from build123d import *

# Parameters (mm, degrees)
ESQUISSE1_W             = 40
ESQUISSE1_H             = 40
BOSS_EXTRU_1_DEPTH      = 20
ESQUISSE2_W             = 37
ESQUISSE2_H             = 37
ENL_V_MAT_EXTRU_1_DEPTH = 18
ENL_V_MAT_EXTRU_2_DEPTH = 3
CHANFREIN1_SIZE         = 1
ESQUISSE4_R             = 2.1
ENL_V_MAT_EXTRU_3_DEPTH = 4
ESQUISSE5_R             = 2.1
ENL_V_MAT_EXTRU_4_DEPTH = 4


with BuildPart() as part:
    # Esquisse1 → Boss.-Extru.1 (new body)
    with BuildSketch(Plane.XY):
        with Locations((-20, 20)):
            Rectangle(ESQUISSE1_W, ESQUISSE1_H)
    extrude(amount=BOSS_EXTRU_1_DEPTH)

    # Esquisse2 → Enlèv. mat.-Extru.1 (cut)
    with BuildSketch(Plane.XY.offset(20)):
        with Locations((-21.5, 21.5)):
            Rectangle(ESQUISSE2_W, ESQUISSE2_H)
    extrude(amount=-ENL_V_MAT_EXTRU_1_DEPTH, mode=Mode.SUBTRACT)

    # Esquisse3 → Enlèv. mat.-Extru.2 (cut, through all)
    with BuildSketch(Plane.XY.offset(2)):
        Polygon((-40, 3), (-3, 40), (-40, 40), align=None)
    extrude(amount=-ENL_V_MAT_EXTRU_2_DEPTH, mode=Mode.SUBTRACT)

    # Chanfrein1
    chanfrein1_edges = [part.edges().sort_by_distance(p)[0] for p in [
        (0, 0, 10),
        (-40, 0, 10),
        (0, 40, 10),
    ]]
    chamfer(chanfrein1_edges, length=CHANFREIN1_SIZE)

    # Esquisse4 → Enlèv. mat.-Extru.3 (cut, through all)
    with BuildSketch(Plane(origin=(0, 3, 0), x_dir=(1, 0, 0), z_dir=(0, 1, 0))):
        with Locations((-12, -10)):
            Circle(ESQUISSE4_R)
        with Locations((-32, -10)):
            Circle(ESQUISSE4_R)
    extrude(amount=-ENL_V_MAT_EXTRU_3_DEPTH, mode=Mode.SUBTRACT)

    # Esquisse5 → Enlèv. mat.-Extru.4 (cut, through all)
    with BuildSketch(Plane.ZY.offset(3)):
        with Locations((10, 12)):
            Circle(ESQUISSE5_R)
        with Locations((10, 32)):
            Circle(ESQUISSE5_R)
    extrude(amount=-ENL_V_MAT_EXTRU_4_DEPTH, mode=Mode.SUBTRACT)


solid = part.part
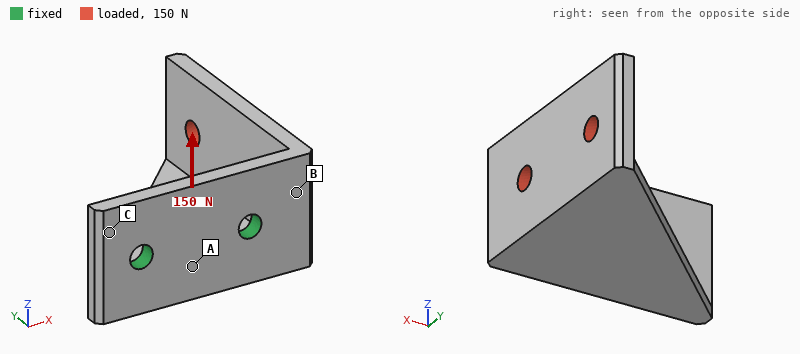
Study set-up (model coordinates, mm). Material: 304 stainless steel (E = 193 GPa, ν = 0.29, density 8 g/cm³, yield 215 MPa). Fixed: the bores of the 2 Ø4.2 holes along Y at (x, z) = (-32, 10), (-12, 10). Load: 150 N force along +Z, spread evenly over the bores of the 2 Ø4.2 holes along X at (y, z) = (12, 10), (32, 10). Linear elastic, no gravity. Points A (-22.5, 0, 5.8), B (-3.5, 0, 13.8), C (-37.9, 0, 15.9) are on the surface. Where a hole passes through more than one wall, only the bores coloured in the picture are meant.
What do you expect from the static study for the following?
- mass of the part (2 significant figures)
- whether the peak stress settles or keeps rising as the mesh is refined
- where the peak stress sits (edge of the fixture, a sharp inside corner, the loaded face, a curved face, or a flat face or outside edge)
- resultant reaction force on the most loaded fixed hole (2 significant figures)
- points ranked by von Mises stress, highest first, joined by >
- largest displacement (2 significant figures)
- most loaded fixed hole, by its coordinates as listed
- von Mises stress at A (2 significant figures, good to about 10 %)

46 g
keeps rising
edge of the fixture
200 N
B > A > C
56 µm
(-12, 10)
18 MPa
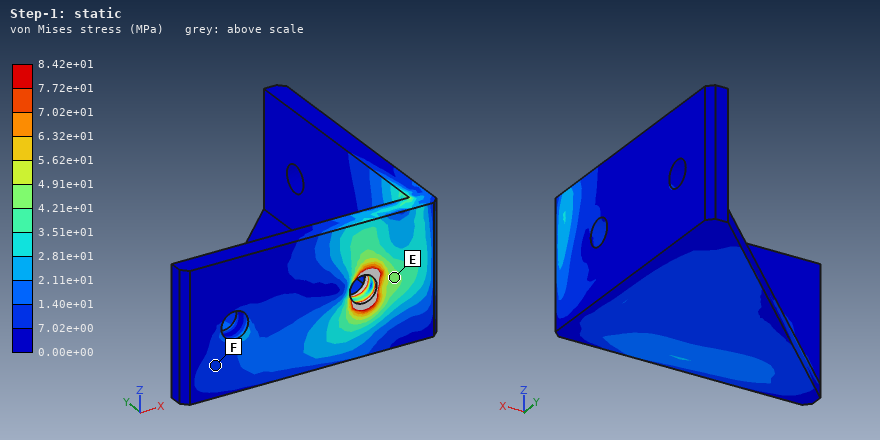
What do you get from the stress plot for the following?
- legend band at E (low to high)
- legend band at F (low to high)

4.21e+01 to 4.91e+01 MPa
7.02e+00 to 1.40e+01 MPa
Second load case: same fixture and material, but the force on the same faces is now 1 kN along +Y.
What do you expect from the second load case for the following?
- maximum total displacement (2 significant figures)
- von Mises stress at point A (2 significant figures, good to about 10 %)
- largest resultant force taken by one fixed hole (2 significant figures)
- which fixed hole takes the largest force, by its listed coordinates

58 µm
25 MPa
1.3 kN
(-12, 10)
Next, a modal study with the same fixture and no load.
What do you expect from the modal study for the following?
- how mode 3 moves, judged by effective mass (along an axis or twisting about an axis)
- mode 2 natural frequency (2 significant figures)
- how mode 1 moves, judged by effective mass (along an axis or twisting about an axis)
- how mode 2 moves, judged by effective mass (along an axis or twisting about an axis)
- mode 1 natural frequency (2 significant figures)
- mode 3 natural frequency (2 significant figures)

along Y
3200 Hz
along Z
along X
2100 Hz
6900 Hz
